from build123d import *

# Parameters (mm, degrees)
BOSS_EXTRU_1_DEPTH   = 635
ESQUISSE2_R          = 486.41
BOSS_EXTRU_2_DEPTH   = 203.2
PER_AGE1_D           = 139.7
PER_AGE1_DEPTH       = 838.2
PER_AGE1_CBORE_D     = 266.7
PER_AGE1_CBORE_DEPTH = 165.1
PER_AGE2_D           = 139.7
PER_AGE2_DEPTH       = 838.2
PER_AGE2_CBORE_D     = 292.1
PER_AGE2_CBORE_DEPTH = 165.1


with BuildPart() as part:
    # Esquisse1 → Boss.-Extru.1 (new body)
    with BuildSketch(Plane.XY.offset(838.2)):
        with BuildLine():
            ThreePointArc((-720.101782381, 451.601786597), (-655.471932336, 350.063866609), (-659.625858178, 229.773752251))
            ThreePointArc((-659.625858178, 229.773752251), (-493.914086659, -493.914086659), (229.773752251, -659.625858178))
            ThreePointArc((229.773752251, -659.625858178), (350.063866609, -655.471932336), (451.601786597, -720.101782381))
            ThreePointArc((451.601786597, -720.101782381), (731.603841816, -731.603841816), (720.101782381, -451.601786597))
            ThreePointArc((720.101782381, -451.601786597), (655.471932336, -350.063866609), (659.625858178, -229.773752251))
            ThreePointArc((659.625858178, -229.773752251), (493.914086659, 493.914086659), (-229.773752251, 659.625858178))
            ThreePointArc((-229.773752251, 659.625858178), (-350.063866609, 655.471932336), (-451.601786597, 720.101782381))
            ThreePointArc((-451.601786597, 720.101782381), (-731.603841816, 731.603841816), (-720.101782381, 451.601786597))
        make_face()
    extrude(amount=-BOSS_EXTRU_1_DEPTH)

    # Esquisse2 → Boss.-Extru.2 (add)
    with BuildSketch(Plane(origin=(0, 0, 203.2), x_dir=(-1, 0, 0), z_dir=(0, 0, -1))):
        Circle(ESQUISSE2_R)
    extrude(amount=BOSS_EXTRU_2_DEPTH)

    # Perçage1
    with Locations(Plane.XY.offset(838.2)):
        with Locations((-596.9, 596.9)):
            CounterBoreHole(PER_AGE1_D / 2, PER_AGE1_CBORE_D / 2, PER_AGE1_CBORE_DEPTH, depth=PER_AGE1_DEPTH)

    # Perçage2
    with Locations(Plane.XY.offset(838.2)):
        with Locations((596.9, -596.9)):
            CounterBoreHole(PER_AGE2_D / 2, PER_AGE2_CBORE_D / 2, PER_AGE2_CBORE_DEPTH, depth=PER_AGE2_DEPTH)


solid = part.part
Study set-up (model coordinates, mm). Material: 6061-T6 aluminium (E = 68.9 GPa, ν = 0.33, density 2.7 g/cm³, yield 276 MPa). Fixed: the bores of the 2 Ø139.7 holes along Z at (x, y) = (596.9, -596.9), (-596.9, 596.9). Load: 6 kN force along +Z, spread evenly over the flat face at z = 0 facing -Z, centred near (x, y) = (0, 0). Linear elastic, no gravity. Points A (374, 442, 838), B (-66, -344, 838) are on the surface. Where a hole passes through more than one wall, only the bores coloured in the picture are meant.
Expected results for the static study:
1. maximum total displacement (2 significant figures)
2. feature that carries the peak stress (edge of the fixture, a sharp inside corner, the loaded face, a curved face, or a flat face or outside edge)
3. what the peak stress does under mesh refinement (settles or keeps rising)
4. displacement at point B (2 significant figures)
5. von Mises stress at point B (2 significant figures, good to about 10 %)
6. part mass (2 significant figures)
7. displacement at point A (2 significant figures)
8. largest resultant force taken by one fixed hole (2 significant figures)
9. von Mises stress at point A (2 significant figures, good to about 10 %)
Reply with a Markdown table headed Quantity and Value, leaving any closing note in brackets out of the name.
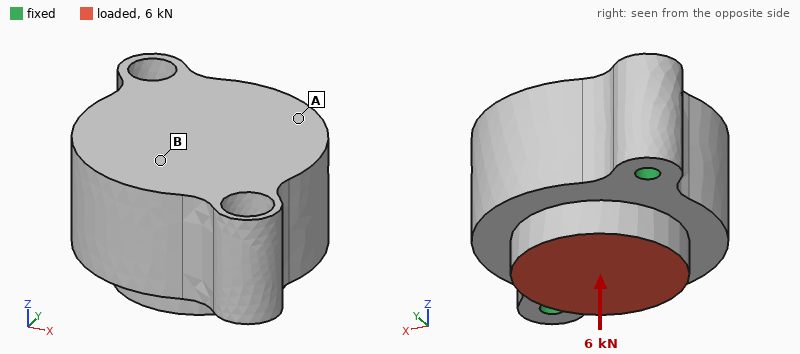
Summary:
| Quantity | Value |
|---|---|
| maximum total displacement | 0.37 µm |
| feature that carries the peak stress | edge of the fixture |
| what the peak stress does under mesh refinement | keeps rising |
| displacement at point B | 0.31 µm |
| von Mises stress at point B | 0.013 MPa |
| part mass | 3400 kg |
| displacement at point A | 0.35 µm |
| largest resultant force taken by one fixed hole | 3.0 kN |
| von Mises stress at point A | 0.0072 MPa |
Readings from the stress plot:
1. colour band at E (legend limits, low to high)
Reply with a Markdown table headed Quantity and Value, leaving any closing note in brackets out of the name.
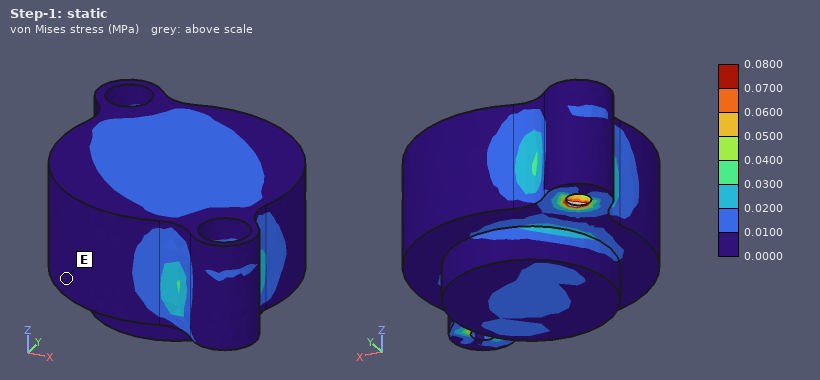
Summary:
| Quantity | Value |
|---|---|
| colour band at E | 0.0000 to 0.0100 MPa |
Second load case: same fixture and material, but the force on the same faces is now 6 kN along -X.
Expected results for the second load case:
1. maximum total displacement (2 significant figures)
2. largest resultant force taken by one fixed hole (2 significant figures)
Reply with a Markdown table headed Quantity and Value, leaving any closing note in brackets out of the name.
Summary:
| Quantity | Value |
|---|---|
| maximum total displacement | 1.3 µm |
| largest resultant force taken by one fixed hole | 3.2 kN |
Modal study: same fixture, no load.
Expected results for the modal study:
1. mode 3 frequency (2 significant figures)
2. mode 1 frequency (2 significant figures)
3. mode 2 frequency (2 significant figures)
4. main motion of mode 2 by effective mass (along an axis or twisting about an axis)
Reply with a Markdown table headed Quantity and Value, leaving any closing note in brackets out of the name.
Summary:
| Quantity | Value |
|---|---|
| mode 3 frequency | 470 Hz |
| mode 1 frequency | 260 Hz |
| mode 2 frequency | 410 Hz |
| main motion of mode 2 by effective mass | along Z |
